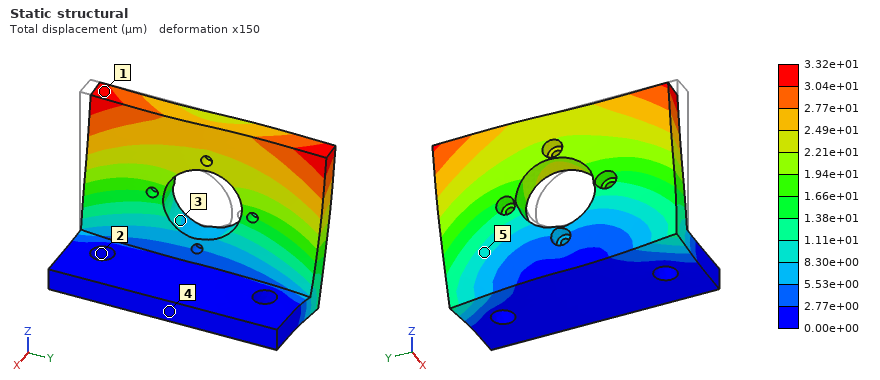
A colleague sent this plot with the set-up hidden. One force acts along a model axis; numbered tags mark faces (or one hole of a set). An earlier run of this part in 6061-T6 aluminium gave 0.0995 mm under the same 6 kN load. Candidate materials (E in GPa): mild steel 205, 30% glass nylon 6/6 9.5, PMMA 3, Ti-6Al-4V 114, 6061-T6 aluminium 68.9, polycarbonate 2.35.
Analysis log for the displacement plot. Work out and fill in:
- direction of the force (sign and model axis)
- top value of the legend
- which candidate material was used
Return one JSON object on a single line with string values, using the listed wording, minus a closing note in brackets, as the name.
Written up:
{"direction of the force": "+Y", "top value of the legend": "3.32e+01 µm", "which candidate material was used": "mild steel"}
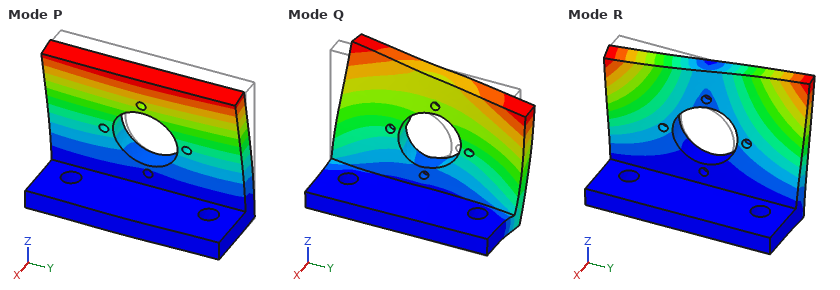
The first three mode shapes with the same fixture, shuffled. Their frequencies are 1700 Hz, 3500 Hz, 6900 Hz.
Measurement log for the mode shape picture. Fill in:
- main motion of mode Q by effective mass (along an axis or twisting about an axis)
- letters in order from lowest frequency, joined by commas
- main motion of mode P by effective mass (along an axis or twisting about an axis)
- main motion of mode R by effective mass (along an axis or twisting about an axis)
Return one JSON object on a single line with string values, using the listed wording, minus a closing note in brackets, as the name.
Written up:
{"main motion of mode Q by effective mass": "along Y", "letters in order from lowest frequency, joined by commas": "P, R, Q", "main motion of mode P by effective mass": "along X", "main motion of mode R by effective mass": "twisting about Z"}
